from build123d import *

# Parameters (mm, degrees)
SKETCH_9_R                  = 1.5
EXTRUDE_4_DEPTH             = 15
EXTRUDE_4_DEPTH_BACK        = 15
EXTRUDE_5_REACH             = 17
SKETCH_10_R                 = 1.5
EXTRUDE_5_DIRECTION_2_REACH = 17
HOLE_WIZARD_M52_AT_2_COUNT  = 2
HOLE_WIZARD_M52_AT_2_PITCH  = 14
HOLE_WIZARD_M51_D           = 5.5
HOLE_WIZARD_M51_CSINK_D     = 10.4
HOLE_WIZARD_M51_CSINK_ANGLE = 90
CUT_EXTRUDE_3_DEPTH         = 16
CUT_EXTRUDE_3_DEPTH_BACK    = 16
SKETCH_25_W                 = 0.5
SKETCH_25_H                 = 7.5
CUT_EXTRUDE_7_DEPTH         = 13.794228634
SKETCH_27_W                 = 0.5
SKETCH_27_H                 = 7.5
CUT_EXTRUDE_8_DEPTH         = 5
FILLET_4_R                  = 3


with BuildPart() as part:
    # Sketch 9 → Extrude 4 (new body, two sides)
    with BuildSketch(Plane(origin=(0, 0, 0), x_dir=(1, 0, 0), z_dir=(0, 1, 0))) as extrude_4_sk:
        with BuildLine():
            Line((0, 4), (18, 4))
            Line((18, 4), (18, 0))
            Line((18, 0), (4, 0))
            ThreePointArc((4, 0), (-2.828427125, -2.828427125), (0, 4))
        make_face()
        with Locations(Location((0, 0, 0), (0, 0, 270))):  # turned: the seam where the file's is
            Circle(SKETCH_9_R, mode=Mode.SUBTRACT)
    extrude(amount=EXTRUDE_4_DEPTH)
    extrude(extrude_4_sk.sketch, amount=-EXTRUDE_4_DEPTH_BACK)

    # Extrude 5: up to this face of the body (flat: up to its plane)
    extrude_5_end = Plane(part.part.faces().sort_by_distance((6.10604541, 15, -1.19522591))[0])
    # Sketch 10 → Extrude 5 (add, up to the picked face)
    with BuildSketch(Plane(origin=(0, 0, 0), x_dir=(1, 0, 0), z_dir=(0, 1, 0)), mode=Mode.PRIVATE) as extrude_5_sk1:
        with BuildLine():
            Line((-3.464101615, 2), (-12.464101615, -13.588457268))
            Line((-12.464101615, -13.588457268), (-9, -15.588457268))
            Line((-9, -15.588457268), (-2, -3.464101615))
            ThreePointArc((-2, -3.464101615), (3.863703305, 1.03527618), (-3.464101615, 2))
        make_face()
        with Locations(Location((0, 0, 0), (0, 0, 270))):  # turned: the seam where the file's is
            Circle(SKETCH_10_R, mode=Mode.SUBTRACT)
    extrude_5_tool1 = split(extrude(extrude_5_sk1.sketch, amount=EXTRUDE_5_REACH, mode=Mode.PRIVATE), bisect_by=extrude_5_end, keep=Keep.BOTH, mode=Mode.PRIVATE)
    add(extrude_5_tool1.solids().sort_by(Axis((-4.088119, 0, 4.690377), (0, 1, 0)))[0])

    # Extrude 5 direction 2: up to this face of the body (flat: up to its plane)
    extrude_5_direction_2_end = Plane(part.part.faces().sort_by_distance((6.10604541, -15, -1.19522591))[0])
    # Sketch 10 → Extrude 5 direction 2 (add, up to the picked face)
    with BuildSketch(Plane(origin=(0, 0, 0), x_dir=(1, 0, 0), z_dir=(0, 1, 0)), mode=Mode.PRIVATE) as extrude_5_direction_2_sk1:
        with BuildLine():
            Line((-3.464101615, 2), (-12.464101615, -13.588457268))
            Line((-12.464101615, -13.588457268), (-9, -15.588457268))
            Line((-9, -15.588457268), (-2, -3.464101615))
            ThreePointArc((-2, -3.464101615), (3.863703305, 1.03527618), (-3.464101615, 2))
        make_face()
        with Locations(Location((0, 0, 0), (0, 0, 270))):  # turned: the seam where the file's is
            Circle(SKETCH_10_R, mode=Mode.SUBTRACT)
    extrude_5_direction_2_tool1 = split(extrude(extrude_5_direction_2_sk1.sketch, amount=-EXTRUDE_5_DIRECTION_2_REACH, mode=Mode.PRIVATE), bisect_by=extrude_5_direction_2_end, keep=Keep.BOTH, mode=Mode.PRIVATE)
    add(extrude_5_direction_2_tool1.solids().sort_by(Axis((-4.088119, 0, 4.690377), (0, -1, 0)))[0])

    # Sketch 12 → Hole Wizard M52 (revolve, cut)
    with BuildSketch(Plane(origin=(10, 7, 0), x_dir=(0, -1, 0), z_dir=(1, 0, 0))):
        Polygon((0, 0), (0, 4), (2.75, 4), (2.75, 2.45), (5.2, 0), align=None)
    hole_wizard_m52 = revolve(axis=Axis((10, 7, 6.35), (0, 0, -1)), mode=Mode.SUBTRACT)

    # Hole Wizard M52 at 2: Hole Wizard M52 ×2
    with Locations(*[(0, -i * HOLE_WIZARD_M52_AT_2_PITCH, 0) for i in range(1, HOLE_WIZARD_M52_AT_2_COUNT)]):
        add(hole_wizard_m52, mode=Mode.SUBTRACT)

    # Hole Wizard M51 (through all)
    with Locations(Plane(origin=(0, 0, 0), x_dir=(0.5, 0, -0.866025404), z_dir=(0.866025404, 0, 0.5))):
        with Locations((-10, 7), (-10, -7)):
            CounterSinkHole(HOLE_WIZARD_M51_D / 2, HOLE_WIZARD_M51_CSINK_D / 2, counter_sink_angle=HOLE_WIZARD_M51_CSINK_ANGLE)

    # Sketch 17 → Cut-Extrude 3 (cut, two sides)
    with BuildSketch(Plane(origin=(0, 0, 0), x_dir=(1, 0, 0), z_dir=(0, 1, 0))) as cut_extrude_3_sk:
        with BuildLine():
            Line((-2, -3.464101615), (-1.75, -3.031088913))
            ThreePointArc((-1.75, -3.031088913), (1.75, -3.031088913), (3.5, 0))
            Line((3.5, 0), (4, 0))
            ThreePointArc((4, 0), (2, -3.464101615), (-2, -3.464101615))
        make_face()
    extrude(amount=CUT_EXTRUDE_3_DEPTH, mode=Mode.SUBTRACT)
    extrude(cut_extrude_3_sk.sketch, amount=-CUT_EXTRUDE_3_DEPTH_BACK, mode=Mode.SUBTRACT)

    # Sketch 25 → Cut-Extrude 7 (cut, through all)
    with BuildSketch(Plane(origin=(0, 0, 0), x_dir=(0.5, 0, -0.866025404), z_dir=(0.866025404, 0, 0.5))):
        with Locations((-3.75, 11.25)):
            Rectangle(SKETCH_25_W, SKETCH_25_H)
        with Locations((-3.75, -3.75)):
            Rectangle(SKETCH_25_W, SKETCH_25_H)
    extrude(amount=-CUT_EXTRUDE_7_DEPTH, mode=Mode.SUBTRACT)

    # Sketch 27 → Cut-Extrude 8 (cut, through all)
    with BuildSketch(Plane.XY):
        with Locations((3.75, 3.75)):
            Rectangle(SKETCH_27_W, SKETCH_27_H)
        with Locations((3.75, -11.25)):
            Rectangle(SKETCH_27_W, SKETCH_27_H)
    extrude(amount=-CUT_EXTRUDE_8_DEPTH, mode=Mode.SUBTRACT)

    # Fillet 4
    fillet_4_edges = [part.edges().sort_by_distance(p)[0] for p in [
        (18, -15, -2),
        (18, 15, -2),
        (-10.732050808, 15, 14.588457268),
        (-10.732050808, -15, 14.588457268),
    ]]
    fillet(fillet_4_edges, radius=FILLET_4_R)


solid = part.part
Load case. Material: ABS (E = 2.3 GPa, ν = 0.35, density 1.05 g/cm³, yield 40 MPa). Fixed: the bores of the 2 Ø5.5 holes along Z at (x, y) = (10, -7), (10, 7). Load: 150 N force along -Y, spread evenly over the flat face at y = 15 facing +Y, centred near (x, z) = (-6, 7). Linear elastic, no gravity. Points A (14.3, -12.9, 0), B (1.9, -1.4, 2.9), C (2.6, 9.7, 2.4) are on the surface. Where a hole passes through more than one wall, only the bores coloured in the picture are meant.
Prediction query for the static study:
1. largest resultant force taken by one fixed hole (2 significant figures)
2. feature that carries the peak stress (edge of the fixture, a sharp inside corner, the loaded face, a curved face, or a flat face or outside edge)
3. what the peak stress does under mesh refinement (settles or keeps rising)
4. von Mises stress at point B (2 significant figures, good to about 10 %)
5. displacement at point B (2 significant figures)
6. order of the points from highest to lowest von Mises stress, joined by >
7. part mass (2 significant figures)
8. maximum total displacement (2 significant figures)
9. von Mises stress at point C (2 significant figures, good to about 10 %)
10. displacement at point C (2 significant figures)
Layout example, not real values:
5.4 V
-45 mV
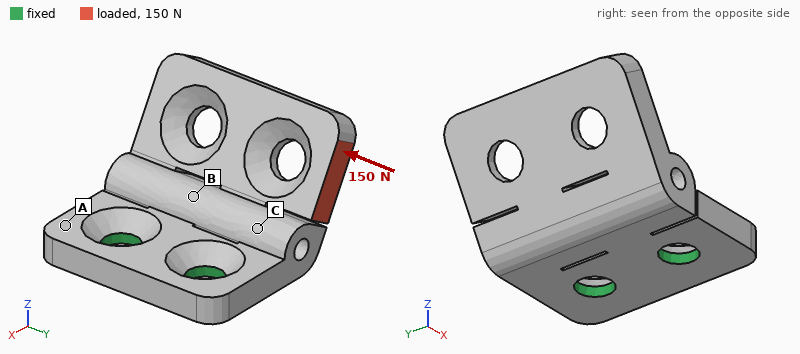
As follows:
190 N
a sharp inside corner
keeps rising
8.2 MPa
0.092 mm
B > C > A
4.2 g
0.49 mm
4.9 MPa
0.13 mm
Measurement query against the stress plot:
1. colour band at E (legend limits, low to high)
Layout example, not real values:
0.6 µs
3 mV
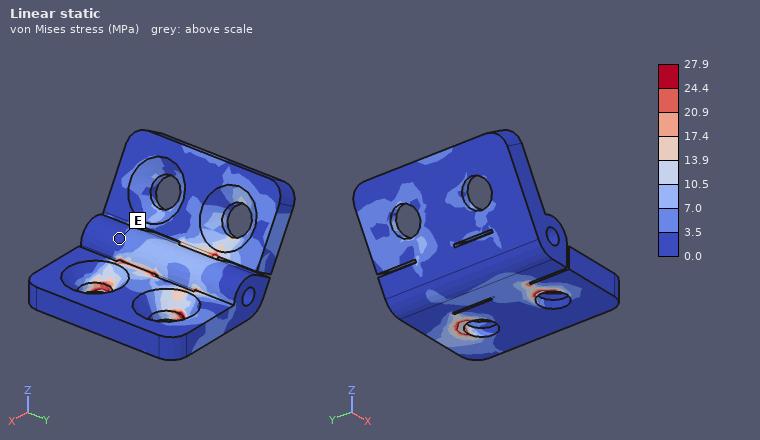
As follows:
0.0 to 3.5 MPa
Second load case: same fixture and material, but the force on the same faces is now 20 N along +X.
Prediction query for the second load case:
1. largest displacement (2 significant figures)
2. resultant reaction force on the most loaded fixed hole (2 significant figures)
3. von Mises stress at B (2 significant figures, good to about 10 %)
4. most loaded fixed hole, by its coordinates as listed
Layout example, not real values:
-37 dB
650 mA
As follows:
0.48 mm
26 N
1.6 MPa
(10, 7)
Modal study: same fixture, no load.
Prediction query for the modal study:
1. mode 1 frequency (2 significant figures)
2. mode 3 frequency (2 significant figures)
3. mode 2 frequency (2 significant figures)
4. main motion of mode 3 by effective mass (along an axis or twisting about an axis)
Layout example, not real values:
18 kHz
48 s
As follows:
900 Hz
3000 Hz
2000 Hz
along Y
